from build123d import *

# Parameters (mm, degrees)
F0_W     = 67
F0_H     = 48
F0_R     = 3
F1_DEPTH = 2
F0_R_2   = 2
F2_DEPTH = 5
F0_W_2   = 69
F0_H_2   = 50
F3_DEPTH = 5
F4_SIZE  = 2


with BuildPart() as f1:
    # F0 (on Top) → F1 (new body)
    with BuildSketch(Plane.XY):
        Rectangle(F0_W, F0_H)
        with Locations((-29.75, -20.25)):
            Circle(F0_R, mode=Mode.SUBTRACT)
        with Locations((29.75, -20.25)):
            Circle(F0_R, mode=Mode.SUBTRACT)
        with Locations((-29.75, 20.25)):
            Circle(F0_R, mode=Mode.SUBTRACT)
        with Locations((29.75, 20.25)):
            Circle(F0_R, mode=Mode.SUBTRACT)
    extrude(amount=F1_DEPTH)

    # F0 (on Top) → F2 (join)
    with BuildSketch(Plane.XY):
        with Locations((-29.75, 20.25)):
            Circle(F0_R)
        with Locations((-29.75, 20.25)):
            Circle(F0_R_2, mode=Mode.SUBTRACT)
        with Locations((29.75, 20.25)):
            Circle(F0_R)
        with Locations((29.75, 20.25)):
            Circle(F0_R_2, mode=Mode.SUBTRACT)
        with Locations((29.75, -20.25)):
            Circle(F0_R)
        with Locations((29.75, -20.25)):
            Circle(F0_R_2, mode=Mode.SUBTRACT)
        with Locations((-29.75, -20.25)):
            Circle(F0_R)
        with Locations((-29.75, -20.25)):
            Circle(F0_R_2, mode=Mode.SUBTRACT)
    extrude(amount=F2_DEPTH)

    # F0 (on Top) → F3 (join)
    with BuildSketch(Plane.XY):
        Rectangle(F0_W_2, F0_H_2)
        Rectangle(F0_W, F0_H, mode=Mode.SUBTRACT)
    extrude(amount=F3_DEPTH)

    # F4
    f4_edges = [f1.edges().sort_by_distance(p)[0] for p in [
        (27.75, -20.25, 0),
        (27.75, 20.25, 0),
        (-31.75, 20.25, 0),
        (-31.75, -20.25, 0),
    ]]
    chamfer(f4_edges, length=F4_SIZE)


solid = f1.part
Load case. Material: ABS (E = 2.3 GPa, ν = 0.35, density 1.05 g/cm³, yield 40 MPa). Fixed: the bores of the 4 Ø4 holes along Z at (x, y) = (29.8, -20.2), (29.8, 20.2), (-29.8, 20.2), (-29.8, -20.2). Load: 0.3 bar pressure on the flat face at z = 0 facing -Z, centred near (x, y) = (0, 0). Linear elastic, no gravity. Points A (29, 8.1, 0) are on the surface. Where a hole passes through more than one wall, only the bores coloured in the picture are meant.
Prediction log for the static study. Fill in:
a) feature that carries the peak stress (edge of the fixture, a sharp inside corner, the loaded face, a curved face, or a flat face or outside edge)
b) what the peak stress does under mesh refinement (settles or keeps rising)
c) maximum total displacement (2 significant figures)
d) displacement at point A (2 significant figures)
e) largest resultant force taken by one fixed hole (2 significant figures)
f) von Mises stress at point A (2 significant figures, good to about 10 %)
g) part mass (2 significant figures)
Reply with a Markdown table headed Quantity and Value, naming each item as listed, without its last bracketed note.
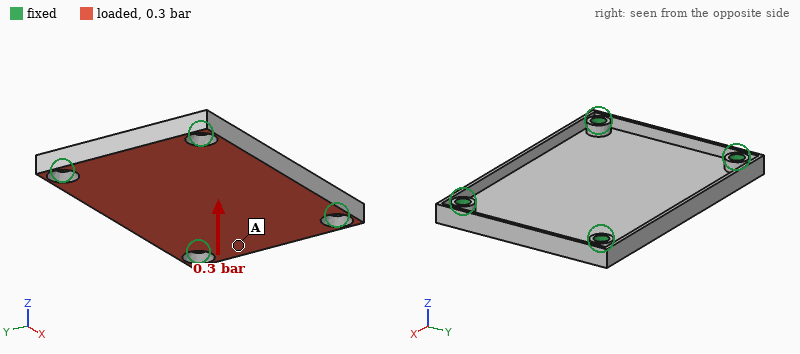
| Quantity | Value |
|---|---|
| feature that carries the peak stress | a sharp inside corner |
| what the peak stress does under mesh refinement | keeps rising |
| maximum total displacement | 0.74 mm |
| displacement at point A | 0.13 mm |
| largest resultant force taken by one fixed hole | 51 N |
| von Mises stress at point A | 3.8 MPa |
| part mass | 7.9 g |
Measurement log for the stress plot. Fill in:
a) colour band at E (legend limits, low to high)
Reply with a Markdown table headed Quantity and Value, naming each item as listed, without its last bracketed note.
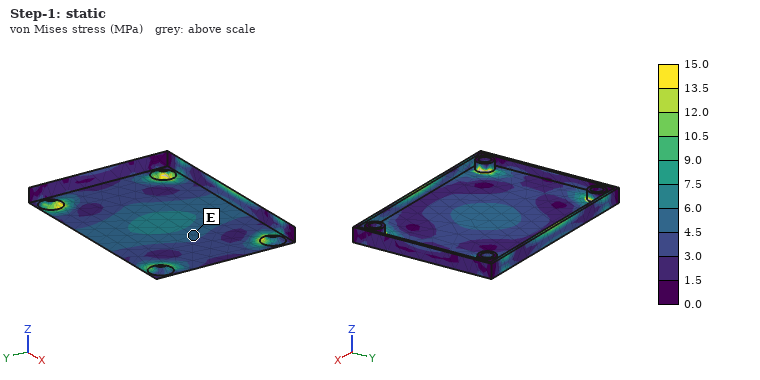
| Quantity | Value |
|---|---|
| colour band at E | 4.5 to 6.0 MPa |
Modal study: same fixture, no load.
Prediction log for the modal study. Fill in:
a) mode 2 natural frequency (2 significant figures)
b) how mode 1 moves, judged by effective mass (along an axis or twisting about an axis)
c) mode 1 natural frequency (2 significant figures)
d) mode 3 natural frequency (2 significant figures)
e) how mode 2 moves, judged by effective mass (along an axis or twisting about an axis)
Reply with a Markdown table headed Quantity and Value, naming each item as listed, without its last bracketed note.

| Quantity | Value |
|---|---|
| mode 2 natural frequency | 1300 Hz |
| how mode 1 moves, judged by effective mass | along Z |
| mode 1 natural frequency | 840 Hz |
| mode 3 natural frequency | 1800 Hz |
| how mode 2 moves, judged by effective mass | twisting about X |
